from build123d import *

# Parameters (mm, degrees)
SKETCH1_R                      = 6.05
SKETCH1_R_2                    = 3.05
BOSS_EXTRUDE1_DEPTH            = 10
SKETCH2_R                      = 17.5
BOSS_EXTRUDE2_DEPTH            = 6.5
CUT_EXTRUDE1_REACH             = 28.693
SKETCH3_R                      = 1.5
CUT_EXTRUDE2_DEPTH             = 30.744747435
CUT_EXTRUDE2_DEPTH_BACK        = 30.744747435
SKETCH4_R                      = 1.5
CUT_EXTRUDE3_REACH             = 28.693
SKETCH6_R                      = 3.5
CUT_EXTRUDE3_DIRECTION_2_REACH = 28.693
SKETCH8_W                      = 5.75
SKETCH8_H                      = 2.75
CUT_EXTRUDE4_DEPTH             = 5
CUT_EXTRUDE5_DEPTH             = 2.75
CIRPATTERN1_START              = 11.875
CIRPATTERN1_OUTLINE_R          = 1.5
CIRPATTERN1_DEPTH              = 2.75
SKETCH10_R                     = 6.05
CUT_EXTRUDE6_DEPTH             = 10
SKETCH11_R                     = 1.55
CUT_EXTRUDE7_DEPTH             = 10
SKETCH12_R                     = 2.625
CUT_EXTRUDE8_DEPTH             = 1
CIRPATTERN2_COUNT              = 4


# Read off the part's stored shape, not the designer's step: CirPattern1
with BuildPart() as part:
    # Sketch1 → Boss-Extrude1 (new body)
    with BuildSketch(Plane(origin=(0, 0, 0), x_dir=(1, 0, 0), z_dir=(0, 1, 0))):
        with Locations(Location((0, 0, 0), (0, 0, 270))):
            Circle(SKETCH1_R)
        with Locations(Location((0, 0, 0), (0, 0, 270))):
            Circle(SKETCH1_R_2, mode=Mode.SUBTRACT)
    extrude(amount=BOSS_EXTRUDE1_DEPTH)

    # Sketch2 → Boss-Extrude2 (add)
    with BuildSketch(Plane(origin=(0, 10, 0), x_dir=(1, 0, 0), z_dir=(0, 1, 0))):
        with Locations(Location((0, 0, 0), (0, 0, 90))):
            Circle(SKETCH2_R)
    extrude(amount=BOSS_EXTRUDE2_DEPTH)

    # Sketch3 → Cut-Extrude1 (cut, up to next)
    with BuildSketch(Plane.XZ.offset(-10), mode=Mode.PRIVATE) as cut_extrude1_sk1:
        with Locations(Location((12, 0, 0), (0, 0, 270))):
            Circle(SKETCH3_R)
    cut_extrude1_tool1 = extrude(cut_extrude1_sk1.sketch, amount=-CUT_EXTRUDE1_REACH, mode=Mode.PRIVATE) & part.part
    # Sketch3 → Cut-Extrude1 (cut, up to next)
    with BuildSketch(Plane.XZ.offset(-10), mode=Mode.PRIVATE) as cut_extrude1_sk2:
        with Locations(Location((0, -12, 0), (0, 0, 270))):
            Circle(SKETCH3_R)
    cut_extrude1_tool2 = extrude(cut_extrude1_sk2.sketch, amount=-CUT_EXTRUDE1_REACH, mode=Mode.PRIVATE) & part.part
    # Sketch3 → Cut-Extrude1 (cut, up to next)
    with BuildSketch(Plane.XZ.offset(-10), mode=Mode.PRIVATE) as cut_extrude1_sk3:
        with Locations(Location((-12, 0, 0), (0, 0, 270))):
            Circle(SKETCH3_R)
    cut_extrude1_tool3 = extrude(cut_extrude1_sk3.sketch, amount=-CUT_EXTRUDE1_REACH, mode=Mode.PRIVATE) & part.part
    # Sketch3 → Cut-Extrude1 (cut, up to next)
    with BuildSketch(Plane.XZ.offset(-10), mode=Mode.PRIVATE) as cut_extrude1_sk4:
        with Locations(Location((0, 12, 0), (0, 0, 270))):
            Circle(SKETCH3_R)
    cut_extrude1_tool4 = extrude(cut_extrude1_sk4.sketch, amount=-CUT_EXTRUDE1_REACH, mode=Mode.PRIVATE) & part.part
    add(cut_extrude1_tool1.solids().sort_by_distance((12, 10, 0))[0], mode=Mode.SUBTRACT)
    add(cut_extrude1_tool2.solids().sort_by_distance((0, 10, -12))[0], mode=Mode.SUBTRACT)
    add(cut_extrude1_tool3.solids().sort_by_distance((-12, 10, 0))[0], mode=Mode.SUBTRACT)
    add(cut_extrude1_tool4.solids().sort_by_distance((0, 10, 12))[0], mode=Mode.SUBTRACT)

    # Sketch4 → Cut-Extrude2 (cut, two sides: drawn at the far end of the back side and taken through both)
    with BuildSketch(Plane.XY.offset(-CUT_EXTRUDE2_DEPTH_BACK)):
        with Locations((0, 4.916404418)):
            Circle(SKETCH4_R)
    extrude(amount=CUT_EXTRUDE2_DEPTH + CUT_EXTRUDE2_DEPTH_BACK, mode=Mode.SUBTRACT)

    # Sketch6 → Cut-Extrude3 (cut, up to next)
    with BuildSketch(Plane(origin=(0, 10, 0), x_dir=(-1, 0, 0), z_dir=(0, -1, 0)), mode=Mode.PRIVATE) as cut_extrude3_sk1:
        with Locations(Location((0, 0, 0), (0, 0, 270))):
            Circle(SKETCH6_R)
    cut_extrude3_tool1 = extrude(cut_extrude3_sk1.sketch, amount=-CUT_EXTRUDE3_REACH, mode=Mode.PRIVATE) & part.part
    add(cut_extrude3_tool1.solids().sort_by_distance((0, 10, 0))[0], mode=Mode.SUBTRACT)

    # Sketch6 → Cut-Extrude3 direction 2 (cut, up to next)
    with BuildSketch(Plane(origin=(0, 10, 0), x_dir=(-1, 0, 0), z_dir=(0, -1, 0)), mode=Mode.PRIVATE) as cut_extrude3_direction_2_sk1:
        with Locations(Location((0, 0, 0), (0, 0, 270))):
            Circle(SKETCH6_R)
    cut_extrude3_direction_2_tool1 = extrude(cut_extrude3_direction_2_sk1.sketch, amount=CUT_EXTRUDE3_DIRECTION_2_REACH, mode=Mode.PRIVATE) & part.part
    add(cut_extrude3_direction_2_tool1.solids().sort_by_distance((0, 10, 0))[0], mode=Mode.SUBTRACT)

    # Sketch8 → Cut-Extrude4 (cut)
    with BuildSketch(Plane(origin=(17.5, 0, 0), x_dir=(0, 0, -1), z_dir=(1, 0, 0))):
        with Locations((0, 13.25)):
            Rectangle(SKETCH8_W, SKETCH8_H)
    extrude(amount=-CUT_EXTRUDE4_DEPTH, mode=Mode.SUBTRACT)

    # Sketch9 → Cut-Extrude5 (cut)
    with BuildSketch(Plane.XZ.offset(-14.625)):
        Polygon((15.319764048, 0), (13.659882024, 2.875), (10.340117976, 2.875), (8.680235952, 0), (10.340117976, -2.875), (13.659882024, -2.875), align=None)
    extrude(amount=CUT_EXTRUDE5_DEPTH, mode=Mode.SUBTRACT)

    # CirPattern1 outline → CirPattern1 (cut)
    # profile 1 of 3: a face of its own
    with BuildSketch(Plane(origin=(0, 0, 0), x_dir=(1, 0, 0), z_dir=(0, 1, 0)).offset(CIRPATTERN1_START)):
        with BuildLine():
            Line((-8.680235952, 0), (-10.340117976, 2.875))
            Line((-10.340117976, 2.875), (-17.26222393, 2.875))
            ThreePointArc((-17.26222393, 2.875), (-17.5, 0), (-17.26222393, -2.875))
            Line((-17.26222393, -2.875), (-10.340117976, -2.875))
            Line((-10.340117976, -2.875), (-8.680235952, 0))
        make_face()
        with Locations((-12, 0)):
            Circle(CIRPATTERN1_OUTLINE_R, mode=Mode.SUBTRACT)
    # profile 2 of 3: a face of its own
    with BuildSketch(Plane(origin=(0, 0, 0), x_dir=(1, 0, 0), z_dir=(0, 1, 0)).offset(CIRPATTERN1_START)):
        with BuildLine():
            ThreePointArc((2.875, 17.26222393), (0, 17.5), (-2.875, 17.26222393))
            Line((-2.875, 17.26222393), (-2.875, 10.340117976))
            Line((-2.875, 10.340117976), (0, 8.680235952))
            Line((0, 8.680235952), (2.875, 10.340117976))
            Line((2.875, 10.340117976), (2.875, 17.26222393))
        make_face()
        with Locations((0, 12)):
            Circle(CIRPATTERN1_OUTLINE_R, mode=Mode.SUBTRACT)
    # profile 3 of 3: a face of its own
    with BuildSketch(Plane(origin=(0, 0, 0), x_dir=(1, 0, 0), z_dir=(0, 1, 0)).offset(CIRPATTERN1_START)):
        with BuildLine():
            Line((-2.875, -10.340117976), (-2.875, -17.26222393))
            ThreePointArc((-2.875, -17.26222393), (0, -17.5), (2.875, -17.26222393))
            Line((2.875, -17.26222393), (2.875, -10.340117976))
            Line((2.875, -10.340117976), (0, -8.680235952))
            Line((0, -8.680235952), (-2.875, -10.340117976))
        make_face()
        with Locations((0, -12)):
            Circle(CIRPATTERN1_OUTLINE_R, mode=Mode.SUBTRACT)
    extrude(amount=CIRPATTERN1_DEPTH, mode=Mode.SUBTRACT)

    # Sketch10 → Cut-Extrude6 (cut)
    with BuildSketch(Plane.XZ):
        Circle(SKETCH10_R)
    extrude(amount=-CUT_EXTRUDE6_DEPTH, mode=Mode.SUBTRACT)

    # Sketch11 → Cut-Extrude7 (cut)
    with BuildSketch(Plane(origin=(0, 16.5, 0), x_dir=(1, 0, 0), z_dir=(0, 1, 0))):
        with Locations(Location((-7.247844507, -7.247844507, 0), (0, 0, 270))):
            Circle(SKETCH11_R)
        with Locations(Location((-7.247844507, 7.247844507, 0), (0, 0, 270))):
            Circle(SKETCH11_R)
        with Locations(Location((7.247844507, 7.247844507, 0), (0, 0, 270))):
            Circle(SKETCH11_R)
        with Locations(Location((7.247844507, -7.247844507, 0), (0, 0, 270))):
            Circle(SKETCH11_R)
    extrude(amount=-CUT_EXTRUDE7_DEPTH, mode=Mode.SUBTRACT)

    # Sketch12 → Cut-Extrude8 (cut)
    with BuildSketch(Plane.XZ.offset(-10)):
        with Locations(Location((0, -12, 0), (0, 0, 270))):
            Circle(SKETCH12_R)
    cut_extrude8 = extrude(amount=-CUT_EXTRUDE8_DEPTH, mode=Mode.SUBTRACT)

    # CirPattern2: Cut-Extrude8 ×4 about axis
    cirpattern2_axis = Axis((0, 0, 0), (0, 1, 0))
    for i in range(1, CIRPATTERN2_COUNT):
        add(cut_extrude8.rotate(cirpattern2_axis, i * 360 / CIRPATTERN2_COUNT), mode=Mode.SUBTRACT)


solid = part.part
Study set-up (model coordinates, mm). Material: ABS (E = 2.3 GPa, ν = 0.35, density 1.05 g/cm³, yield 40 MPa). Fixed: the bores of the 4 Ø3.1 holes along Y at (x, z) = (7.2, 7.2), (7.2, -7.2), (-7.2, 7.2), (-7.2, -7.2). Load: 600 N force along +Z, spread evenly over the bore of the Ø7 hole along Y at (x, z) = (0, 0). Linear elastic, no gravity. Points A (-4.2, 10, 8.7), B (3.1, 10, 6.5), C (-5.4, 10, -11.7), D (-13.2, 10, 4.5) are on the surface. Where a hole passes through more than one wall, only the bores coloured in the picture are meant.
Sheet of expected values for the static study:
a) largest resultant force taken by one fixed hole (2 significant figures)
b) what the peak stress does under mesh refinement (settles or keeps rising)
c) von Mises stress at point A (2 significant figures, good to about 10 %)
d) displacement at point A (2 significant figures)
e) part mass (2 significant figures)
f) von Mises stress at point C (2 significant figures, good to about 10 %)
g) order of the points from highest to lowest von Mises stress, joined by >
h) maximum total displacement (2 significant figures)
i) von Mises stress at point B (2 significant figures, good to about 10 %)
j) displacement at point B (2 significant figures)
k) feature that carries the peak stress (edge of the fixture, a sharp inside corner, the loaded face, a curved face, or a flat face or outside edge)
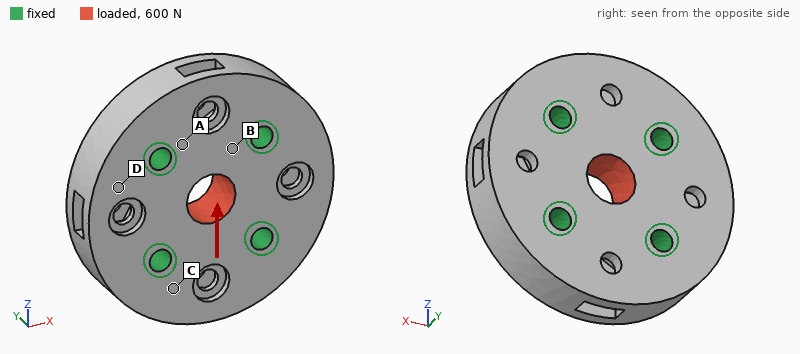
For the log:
160 N
keeps rising
2.2 MPa
4.9 µm
5.4 g
1.4 MPa
B > A > C > D
17 µm
3.2 MPa
8.2 µm
edge of the fixture
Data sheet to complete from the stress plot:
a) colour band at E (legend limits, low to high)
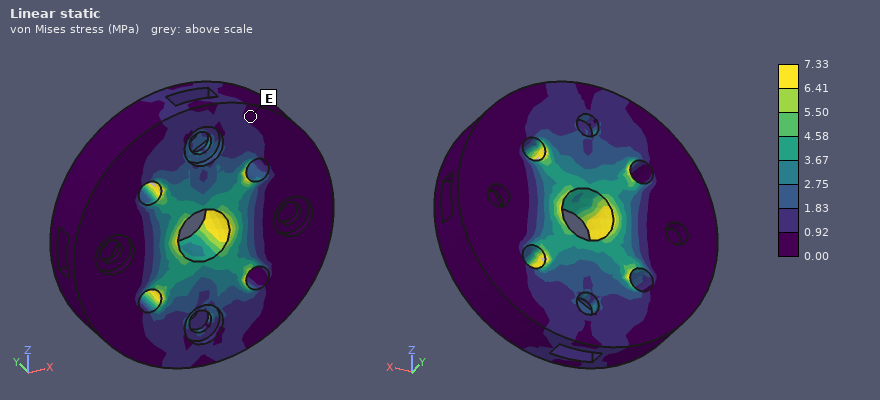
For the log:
0.00 to 0.92 MPa
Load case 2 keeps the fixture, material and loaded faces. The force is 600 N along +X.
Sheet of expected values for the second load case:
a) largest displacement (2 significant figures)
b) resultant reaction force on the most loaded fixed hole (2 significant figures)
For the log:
17 µm
160 N
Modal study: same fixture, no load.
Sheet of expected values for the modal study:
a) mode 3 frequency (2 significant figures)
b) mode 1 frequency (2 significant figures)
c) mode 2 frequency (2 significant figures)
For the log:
14 kHz
13 kHz
14 kHz
